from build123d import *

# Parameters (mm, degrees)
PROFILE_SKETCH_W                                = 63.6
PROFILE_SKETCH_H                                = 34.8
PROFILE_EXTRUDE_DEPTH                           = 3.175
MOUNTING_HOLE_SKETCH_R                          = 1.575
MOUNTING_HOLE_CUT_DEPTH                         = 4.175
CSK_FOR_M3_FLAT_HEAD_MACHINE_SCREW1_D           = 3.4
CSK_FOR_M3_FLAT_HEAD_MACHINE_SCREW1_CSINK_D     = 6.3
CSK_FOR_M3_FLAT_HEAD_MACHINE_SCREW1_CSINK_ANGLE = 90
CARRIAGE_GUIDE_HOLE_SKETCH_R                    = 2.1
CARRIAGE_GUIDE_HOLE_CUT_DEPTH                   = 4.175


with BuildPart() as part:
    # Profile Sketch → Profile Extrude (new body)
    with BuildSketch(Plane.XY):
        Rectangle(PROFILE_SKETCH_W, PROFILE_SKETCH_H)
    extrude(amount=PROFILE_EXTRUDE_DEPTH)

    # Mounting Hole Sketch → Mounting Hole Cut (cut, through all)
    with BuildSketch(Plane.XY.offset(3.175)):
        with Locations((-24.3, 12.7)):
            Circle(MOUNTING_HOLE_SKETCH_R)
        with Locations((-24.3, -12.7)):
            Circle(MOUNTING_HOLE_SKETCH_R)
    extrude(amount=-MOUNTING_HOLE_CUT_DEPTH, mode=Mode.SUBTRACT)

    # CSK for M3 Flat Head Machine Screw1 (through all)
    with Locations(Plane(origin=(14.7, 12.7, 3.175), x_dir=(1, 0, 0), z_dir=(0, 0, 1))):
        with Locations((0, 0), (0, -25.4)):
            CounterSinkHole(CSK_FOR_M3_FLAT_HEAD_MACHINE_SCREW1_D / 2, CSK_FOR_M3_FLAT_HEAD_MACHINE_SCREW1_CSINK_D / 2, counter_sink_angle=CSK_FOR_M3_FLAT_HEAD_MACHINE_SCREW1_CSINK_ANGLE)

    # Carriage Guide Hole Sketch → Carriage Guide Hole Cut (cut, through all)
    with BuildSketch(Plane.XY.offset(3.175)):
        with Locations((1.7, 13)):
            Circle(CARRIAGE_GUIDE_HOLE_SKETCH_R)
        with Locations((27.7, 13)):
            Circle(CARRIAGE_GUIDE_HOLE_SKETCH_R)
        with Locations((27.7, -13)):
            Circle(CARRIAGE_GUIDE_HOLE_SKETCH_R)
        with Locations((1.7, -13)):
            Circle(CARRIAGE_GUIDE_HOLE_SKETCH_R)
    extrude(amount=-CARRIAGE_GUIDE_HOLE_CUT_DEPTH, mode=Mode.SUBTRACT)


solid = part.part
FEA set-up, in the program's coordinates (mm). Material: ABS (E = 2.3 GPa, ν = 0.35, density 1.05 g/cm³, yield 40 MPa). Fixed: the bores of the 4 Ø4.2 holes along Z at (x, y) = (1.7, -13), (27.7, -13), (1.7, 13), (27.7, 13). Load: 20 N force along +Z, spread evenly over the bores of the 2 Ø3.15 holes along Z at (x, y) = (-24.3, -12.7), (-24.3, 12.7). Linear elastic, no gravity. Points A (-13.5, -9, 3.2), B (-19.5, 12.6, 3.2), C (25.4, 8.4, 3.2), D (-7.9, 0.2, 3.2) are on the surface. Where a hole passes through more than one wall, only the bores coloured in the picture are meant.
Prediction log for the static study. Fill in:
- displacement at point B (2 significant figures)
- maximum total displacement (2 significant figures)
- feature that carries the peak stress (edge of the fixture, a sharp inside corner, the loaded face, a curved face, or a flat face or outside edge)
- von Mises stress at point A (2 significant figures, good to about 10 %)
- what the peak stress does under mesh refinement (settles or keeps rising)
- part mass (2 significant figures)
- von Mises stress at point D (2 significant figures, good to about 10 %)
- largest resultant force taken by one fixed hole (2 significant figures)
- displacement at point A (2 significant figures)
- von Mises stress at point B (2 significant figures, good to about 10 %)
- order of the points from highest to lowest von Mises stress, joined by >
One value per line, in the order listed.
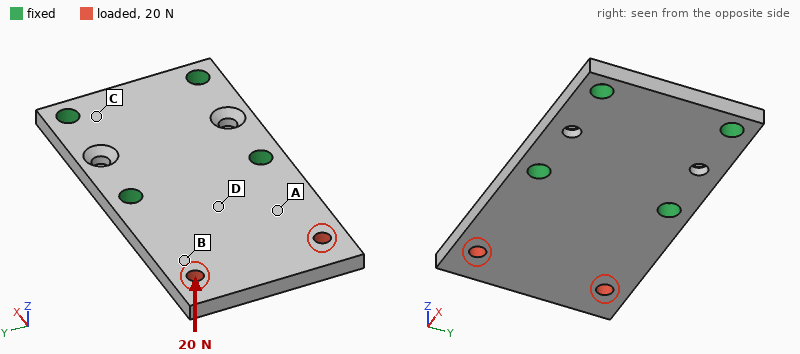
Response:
0.38 mm
0.75 mm
edge of the fixture
3.5 MPa
keeps rising
7.1 g
4.7 MPa
12 N
0.22 mm
2.0 MPa
D > A > B > C
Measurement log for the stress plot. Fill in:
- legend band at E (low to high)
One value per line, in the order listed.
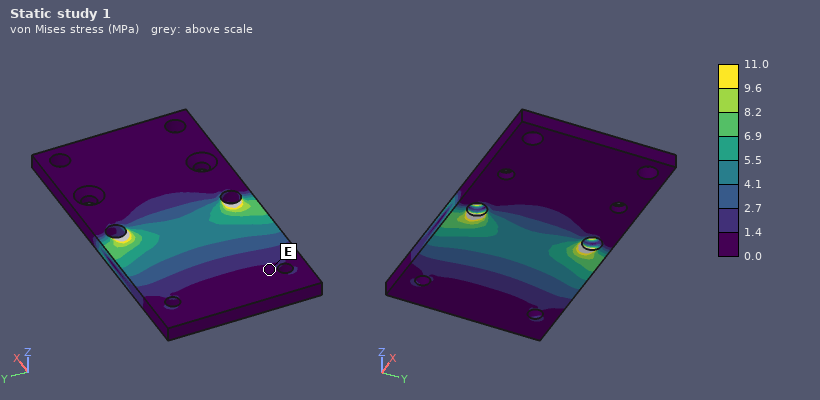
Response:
0.0 to 1.4 MPa
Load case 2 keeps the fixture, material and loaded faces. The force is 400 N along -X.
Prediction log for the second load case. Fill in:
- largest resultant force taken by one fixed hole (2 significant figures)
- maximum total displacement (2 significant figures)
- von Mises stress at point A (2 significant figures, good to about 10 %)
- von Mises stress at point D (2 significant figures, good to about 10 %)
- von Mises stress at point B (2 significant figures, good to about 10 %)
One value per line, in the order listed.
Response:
180 N
64 µm
3.6 MPa
2.0 MPa
5.9 MPa
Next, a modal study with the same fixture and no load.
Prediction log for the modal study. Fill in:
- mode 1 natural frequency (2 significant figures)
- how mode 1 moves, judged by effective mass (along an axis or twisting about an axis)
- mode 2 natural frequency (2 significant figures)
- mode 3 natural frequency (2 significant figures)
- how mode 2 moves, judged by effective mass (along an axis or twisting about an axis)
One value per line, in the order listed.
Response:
690 Hz
along Z
1700 Hz
4000 Hz
twisting about X
